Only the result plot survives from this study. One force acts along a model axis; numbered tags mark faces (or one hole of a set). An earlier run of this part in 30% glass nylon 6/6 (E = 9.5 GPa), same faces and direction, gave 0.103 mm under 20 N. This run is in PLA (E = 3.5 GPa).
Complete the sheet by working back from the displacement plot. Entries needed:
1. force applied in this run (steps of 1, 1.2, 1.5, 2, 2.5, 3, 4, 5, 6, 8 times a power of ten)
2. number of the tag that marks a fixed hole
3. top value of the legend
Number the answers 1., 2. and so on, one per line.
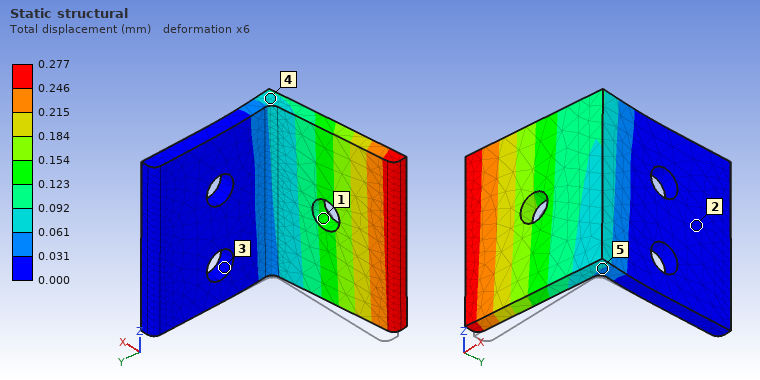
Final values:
1. 20 N
2. 3
3. 0.277 mm
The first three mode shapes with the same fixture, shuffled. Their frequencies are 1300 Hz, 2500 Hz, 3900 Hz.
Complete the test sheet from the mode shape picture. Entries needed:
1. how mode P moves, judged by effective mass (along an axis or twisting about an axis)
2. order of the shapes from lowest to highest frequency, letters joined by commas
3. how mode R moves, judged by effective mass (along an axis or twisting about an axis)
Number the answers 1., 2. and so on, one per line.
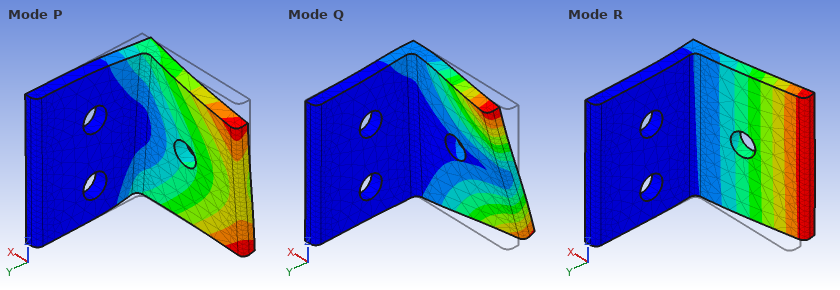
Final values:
1. along Z
2. R, P, Q
3. along Y
